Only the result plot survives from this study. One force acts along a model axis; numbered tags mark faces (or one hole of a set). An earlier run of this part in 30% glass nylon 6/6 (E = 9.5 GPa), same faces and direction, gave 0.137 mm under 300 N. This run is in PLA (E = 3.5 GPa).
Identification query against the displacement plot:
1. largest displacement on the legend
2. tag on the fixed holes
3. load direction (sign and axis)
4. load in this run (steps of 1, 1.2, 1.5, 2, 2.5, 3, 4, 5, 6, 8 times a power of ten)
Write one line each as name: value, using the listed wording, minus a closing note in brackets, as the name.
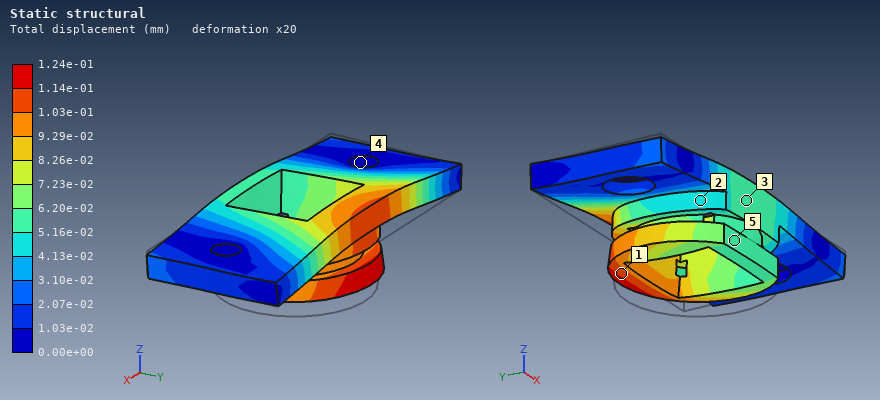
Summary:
largest displacement on the legend: 1.24e-01 mm
tag on the fixed holes: 4
load direction: +Z
load in this run: 100 N
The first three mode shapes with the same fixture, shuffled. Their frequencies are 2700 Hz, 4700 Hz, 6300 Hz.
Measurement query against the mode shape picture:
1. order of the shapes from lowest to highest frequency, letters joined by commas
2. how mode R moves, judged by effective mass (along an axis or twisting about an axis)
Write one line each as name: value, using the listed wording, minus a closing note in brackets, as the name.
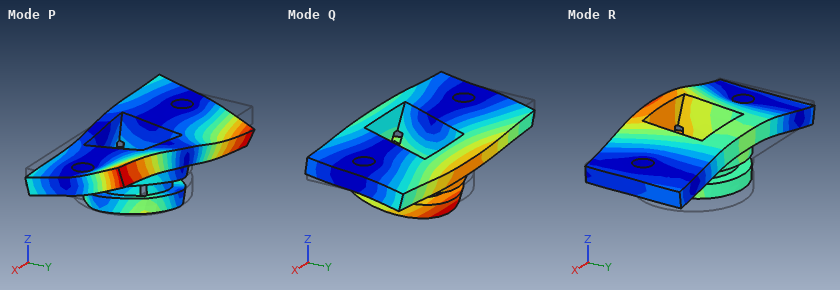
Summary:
order of the shapes from lowest to highest frequency, letters joined by commas: Q, R, P
how mode R moves, judged by effective mass: along Z
